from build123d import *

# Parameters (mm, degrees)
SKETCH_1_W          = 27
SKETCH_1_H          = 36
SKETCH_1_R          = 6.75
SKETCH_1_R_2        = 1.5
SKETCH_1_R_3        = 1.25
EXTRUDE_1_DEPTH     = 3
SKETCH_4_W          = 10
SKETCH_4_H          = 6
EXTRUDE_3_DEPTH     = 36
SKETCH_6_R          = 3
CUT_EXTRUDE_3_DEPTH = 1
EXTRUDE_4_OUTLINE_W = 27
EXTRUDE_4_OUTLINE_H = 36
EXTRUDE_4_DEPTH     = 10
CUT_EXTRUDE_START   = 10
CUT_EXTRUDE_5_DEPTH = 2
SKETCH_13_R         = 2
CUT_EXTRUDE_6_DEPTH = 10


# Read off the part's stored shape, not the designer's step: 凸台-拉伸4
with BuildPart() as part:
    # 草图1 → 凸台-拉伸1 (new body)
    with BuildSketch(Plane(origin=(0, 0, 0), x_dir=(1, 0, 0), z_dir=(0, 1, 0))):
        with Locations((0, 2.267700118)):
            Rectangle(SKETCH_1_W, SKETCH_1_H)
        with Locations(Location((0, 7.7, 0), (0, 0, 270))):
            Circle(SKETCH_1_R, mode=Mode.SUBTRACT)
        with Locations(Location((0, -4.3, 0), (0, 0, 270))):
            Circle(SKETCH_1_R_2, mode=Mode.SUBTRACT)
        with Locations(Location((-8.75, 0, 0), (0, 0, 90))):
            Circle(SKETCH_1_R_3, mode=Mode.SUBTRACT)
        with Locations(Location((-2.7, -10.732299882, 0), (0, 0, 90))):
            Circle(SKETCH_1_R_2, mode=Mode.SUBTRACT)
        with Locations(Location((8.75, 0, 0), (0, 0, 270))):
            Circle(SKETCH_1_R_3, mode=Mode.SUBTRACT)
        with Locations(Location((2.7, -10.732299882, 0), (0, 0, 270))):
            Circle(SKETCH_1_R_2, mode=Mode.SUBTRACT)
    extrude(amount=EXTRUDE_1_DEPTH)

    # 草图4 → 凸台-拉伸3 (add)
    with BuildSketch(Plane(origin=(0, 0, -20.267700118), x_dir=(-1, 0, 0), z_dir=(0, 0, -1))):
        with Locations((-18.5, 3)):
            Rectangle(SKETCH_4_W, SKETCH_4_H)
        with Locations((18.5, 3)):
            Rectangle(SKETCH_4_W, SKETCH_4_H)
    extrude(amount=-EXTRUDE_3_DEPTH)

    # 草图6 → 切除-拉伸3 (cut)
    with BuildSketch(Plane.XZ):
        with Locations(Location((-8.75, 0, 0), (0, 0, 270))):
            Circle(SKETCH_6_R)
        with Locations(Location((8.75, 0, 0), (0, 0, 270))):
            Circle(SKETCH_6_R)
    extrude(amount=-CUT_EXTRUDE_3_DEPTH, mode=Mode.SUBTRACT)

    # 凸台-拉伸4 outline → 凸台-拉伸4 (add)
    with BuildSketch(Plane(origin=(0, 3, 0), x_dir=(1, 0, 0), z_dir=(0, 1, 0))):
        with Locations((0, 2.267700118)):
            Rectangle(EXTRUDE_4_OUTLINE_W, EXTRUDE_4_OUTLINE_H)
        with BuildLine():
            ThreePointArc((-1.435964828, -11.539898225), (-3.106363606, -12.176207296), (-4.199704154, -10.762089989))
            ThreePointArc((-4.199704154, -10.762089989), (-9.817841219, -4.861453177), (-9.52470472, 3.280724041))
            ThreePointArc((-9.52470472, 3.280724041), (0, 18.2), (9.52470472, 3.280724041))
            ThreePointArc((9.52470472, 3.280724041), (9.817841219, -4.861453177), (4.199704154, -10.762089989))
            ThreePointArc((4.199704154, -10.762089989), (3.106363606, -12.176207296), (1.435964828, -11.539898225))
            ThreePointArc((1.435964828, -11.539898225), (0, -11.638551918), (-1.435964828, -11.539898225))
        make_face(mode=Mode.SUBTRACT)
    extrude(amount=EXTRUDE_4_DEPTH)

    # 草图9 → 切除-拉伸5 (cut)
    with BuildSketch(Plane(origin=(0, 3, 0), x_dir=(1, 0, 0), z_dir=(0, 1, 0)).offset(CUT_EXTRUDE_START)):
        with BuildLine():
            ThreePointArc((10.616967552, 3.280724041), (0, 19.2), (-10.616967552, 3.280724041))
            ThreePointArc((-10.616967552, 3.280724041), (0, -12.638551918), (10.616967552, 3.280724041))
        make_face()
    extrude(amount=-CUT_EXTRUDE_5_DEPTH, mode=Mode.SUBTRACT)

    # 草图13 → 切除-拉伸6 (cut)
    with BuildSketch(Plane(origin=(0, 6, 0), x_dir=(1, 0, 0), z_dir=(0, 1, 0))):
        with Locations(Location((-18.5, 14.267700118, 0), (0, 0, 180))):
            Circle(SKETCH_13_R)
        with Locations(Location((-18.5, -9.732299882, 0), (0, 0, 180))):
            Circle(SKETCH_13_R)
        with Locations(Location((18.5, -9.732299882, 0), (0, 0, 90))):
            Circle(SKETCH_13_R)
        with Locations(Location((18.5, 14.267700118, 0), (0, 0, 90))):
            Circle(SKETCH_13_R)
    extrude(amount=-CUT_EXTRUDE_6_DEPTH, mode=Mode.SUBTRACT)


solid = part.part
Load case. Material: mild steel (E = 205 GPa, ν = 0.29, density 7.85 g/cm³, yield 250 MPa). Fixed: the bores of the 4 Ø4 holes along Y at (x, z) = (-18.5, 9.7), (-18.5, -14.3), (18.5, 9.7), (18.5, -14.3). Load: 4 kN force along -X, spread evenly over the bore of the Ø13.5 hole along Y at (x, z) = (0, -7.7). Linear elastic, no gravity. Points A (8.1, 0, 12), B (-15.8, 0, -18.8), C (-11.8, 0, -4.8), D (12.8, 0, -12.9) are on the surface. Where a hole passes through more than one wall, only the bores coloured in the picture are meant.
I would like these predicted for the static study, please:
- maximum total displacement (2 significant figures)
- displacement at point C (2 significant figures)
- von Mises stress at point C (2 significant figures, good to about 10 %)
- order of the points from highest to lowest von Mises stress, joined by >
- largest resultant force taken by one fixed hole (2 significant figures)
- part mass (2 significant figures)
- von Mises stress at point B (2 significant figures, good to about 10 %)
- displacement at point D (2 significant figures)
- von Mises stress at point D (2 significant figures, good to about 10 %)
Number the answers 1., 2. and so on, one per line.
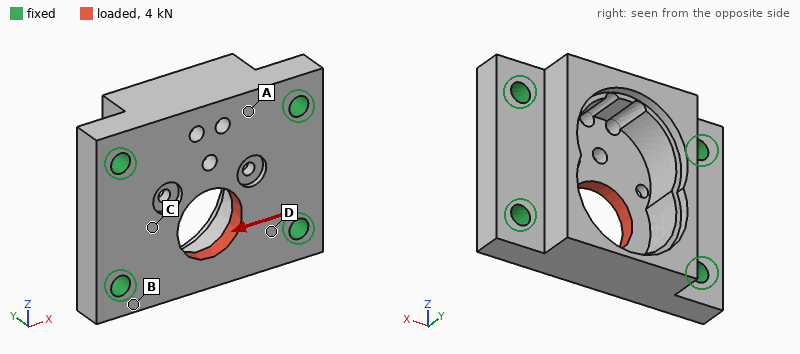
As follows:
1. 2.8 µm
2. 1.5 µm
3. 25 MPa
4. D > C > B > A
5. 1.4 kN
6. 83 g
7. 11 MPa
8. 0.71 µm
9. 35 MPa
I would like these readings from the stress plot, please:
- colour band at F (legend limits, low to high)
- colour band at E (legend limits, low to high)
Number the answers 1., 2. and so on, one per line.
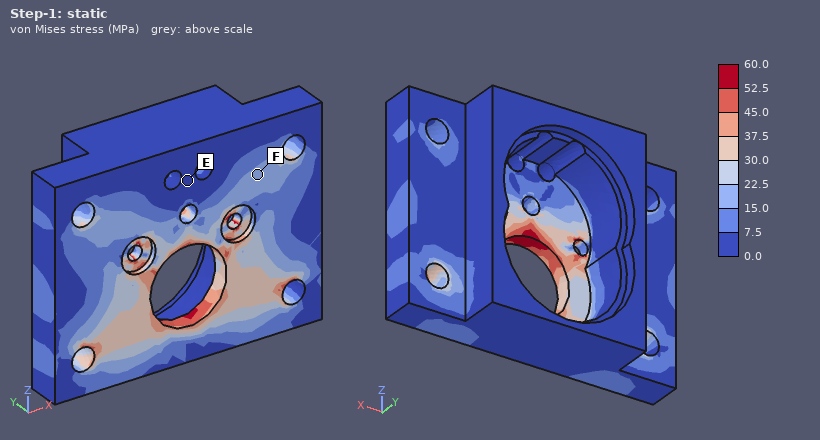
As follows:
1. 15.0 to 22.5 MPa
2. 0.0 to 7.5 MPa
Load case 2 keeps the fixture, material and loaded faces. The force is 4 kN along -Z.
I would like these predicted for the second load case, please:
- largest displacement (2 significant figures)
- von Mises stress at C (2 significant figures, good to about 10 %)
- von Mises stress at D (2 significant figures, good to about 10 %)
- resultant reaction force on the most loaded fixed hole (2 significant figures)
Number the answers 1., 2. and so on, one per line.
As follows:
1. 6.2 µm
2. 28 MPa
3. 25 MPa
4. 1.1 kN
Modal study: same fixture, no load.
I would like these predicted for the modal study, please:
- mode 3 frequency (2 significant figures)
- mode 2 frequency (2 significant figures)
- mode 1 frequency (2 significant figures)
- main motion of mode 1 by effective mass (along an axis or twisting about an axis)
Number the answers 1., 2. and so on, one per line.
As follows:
1. 31 kHz
2. 23 kHz
3. 21 kHz
4. along Y
